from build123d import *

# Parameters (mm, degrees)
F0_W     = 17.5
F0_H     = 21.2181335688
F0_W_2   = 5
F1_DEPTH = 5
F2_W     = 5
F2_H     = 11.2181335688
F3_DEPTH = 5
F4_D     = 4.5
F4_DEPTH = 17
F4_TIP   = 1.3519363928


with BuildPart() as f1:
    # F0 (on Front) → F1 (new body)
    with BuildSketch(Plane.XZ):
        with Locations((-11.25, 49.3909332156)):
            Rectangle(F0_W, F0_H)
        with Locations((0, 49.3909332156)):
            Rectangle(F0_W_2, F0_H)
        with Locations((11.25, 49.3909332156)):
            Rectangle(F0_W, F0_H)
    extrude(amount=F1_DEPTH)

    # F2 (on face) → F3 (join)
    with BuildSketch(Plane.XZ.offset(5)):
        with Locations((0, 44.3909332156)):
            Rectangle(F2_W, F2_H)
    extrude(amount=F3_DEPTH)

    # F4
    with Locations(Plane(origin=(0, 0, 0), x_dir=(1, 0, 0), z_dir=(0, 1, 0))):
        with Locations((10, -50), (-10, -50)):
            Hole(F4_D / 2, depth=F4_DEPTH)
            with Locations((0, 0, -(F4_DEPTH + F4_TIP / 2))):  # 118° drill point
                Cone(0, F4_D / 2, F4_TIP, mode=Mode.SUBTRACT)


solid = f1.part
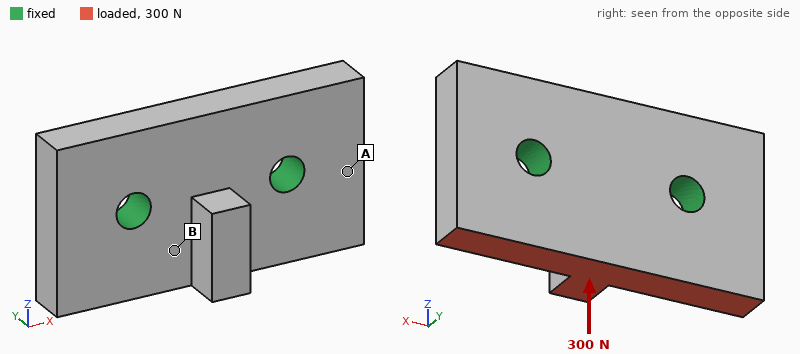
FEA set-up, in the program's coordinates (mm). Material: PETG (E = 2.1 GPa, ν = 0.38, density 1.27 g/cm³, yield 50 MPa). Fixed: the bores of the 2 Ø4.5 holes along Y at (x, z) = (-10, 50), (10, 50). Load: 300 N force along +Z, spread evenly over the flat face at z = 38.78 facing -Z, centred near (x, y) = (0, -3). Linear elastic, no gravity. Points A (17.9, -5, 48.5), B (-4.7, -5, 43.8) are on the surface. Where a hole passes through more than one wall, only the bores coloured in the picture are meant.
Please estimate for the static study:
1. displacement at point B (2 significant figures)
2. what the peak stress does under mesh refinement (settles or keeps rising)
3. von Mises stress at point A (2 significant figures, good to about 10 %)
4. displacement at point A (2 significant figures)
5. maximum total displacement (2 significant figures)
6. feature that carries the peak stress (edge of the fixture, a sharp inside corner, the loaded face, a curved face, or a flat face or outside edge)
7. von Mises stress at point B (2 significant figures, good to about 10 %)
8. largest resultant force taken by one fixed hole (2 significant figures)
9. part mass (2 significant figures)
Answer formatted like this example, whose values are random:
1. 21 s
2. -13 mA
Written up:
1. 11 µm
2. keeps rising
3. 0.92 MPa
4. 8.0 µm
5. 30 µm
6. edge of the fixture
7. 2.2 MPa
8. 150 N
9. 5.5 g
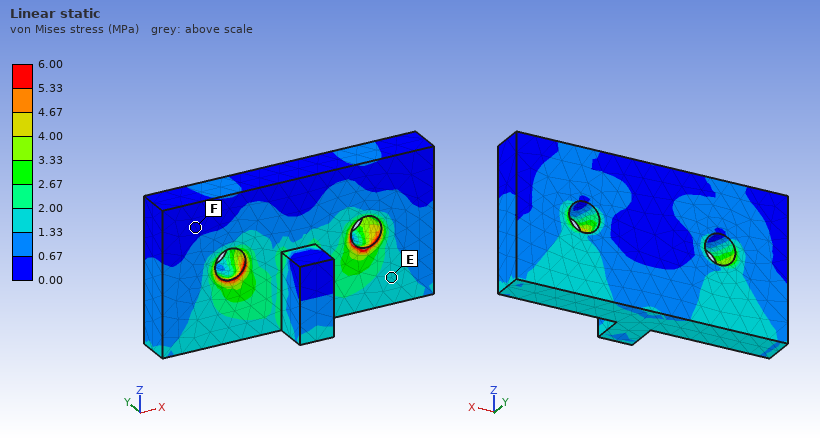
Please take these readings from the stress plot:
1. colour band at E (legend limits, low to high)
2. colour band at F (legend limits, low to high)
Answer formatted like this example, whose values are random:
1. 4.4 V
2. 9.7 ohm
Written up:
1. 1.33 to 2.00 MPa
2. 0.00 to 0.67 MPa
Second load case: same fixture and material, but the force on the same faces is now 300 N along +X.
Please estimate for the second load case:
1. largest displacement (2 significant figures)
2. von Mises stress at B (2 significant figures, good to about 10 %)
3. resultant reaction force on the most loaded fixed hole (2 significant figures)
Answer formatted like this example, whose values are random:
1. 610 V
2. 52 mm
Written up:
1. 54 µm
2. 4.7 MPa
3. 200 N
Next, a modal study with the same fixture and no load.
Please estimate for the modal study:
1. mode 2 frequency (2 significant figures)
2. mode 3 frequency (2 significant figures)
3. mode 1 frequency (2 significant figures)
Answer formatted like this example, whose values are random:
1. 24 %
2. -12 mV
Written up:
1. 7400 Hz
2. 7900 Hz
3. 6200 Hz
